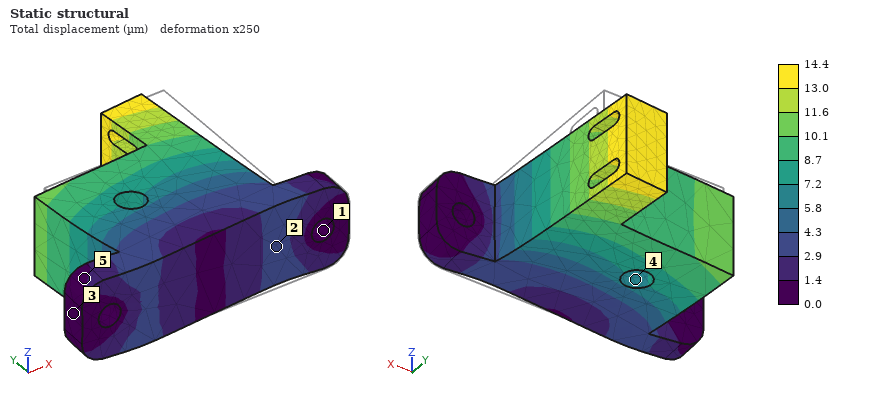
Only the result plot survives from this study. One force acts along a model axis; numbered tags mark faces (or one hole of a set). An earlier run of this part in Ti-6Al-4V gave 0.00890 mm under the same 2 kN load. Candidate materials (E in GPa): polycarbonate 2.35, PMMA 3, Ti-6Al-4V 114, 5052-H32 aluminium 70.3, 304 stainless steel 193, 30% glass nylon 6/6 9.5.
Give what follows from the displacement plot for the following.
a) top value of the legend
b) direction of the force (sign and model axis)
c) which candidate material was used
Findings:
14.4 µm
-X
5052-H32 aluminium
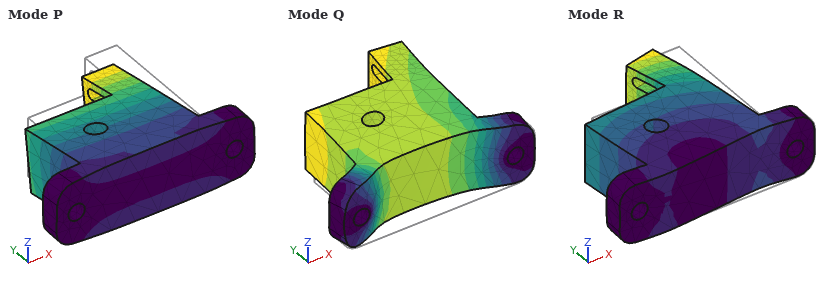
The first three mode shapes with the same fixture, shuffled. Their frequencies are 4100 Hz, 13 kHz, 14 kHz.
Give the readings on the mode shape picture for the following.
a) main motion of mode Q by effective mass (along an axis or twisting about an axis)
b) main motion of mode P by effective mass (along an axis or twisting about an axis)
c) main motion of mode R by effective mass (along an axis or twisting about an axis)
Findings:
along Y
along Z
along X
